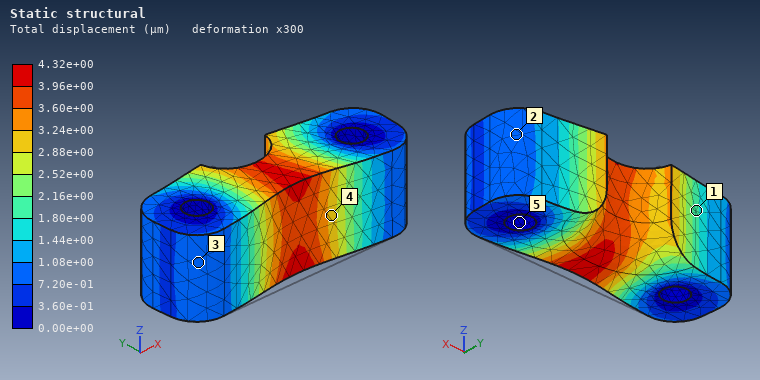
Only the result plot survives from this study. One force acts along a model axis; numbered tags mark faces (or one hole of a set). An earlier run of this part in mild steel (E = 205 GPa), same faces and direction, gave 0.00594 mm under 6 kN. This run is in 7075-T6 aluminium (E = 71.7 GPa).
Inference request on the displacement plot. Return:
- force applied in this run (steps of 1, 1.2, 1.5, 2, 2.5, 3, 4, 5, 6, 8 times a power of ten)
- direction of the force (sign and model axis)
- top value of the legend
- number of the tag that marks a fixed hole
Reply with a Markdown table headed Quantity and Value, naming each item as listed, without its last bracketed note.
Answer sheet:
| Quantity | Value |
|---|---|
| force applied in this run | 1.5 kN |
| direction of the force | +Y |
| top value of the legend | 4.32e+00 µm |
| number of the tag that marks a fixed hole | 5 |
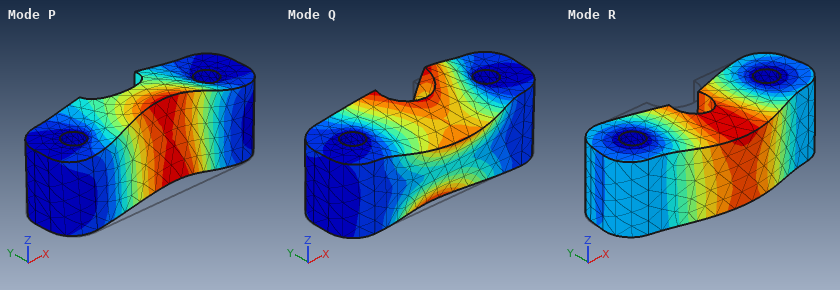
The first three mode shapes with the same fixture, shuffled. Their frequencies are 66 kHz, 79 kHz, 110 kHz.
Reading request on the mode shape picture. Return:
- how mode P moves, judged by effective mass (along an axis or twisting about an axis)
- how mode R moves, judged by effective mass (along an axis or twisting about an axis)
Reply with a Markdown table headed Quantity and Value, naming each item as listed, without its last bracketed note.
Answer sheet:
| Quantity | Value |
|---|---|
| how mode P moves, judged by effective mass | along Z |
| how mode R moves, judged by effective mass | along Y |
